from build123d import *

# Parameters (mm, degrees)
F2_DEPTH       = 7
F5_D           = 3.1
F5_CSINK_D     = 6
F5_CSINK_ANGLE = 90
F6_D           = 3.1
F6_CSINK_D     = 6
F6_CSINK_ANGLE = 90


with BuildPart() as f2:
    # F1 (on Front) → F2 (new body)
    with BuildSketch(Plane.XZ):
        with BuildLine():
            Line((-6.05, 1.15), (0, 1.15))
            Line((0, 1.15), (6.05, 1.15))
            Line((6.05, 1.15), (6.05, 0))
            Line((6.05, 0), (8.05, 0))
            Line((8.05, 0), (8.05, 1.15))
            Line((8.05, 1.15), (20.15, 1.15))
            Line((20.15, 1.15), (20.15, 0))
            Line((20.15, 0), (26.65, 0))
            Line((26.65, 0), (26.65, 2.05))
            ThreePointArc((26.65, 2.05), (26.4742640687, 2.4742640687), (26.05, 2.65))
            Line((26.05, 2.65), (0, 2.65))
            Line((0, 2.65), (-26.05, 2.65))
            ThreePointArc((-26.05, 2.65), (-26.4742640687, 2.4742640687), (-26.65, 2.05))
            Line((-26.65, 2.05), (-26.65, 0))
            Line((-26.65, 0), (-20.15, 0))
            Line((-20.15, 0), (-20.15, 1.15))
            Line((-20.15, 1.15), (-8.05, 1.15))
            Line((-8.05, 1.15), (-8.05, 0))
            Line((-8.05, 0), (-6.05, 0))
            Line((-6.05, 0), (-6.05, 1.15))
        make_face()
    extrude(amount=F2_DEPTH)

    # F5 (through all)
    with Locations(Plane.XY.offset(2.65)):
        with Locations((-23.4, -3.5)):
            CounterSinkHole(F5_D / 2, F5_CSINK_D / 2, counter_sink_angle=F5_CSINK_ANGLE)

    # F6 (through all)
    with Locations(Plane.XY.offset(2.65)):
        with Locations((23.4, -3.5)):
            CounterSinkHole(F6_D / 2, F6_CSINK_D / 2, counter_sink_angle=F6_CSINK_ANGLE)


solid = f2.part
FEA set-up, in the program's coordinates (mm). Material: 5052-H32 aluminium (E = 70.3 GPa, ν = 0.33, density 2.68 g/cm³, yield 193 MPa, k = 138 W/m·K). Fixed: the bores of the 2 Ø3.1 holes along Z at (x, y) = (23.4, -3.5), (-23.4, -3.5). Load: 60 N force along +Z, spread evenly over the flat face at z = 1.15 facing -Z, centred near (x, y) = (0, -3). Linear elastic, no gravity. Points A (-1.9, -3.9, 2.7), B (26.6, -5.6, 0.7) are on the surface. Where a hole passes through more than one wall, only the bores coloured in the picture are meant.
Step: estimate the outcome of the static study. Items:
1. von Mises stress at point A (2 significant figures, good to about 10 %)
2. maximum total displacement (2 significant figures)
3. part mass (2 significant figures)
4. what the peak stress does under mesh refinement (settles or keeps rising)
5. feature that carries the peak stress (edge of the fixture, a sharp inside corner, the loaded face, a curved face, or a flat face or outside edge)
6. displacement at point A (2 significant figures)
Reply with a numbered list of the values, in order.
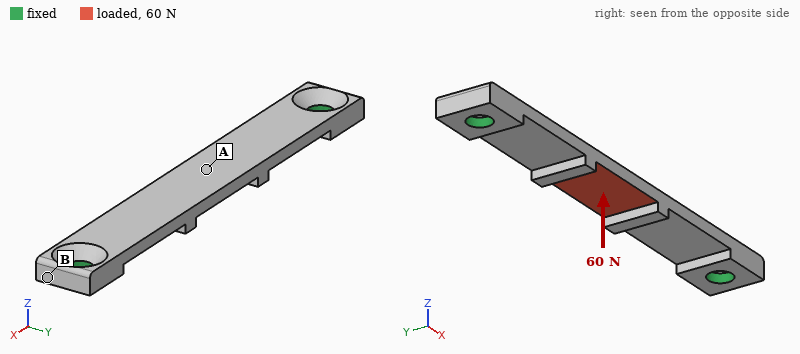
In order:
1. 92 MPa
2. 0.17 mm
3. 1.7 g
4. keeps rising
5. edge of the fixture
6. 0.16 mm
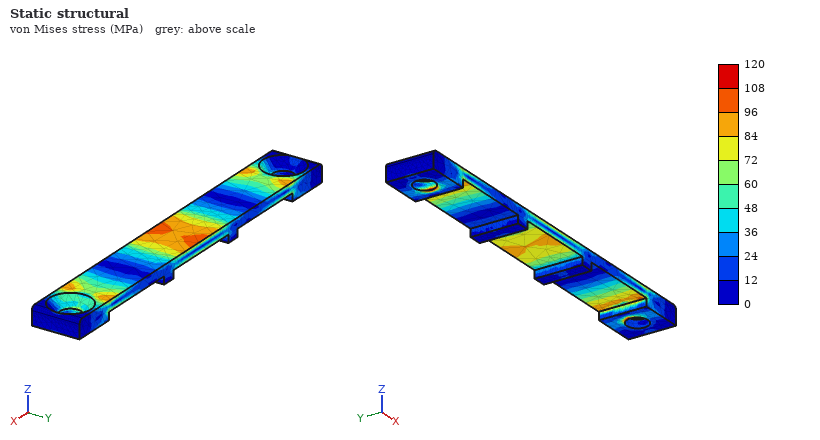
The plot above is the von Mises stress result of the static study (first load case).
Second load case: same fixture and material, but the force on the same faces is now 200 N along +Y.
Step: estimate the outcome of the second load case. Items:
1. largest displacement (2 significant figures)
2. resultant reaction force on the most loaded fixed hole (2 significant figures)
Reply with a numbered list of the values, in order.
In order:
1. 58 µm
2. 100 N
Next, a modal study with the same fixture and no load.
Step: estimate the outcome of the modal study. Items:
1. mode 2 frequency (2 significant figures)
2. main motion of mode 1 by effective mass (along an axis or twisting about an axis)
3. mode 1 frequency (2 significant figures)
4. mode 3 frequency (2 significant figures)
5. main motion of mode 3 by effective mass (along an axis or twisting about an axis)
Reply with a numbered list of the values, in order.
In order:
1. 11 kHz
2. along Z
3. 4000 Hz
4. 13 kHz
5. along Y
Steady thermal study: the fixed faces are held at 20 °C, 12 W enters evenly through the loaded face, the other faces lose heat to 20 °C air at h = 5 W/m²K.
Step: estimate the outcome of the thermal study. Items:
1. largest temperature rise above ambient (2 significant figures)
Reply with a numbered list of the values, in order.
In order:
1. 79 K
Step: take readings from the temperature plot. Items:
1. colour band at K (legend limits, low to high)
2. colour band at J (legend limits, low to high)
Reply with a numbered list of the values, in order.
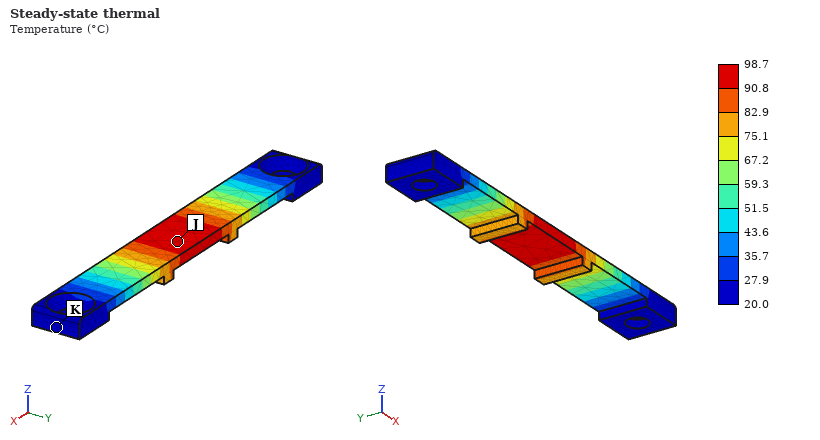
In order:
1. 20.0 to 27.9 °C
2. 90.8 to 98.7 °C
